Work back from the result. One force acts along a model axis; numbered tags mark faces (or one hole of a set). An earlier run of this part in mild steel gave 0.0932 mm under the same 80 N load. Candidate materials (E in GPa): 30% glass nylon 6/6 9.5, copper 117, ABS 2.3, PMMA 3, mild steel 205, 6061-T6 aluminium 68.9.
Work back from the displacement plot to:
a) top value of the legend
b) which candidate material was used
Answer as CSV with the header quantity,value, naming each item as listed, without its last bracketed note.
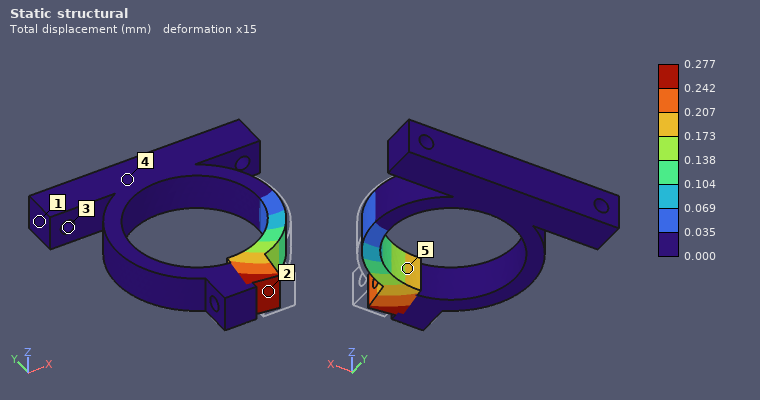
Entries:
quantity,value
top value of the legend,0.277 mm
which candidate material was used,6061-T6 aluminium
